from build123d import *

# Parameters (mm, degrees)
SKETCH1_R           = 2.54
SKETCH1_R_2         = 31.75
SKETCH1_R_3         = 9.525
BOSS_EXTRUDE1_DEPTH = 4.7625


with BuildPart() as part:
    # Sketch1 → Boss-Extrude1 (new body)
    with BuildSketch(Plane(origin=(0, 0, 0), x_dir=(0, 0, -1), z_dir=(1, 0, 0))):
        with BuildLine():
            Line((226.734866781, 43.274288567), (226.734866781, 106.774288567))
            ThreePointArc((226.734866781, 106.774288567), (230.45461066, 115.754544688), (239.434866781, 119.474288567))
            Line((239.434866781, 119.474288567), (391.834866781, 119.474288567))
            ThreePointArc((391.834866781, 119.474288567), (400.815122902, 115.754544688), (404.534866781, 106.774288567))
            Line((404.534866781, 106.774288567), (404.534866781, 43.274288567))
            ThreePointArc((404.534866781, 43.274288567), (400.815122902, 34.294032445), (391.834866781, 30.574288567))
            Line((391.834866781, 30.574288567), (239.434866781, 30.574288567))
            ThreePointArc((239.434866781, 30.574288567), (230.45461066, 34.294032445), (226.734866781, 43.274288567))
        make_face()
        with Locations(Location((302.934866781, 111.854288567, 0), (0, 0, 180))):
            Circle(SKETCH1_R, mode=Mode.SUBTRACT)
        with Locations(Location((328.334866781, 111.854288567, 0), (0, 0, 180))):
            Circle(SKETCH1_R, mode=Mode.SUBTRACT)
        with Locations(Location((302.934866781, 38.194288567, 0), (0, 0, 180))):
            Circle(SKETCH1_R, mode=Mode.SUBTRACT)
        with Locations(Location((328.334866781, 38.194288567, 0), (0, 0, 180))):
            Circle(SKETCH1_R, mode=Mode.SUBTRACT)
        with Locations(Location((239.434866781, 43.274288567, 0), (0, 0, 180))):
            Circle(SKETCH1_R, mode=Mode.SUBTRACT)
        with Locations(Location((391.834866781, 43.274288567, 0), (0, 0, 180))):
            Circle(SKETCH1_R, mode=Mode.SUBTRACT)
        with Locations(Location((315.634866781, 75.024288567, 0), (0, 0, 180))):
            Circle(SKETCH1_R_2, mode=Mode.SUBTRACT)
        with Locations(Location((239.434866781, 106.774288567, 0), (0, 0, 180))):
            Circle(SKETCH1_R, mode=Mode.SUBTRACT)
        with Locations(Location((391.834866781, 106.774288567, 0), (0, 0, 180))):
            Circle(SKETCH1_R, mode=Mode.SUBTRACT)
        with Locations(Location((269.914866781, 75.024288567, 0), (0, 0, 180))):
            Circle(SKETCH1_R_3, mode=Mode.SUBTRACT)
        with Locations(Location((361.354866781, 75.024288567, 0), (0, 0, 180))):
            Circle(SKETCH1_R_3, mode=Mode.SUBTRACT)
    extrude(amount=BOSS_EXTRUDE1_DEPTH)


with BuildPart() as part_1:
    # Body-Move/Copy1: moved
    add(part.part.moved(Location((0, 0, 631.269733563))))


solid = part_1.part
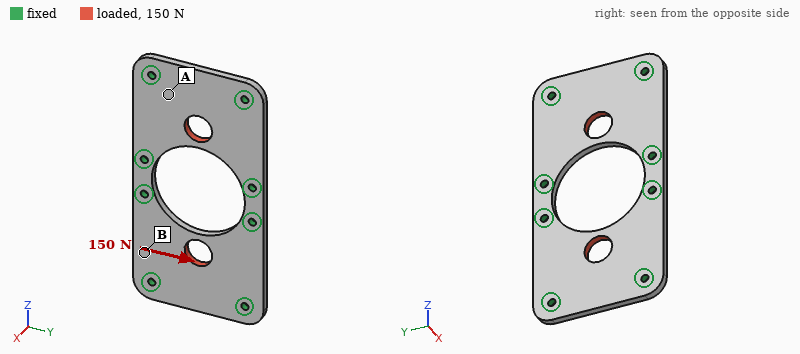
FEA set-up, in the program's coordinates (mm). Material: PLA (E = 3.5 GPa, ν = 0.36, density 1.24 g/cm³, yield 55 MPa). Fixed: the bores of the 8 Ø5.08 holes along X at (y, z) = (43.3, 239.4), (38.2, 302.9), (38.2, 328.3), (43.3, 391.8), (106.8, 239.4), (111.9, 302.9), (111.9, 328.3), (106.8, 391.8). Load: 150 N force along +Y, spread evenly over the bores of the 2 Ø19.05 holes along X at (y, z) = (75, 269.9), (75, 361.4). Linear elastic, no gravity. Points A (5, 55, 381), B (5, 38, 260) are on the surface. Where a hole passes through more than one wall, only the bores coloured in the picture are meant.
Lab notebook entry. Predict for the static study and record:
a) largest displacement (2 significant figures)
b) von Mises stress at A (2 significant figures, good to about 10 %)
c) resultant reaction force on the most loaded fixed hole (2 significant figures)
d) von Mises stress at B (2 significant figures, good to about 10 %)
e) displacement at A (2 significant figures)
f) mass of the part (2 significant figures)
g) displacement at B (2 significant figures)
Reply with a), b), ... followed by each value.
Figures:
a) 4.6 µm
b) 0.28 MPa
c) 29 N
d) 0.11 MPa
e) 1.6 µm
f) 70 g
g) 2.7 µm
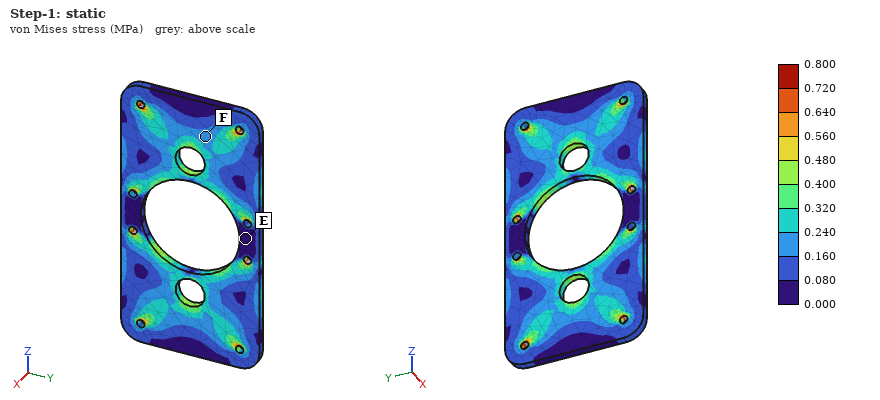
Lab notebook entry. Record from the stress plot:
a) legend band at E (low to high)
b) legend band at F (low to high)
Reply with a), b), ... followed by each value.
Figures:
a) 0.000 to 0.080 MPa
b) 0.160 to 0.240 MPa
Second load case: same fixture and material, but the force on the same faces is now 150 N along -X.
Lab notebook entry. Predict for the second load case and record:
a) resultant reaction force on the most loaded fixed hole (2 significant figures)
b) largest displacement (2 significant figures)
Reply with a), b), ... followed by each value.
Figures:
a) 22 N
b) 0.24 mm
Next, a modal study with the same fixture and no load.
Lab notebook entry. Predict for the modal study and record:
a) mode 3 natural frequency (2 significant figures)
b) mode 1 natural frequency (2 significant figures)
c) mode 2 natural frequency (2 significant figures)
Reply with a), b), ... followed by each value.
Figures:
a) 2100 Hz
b) 1300 Hz
c) 1300 Hz
